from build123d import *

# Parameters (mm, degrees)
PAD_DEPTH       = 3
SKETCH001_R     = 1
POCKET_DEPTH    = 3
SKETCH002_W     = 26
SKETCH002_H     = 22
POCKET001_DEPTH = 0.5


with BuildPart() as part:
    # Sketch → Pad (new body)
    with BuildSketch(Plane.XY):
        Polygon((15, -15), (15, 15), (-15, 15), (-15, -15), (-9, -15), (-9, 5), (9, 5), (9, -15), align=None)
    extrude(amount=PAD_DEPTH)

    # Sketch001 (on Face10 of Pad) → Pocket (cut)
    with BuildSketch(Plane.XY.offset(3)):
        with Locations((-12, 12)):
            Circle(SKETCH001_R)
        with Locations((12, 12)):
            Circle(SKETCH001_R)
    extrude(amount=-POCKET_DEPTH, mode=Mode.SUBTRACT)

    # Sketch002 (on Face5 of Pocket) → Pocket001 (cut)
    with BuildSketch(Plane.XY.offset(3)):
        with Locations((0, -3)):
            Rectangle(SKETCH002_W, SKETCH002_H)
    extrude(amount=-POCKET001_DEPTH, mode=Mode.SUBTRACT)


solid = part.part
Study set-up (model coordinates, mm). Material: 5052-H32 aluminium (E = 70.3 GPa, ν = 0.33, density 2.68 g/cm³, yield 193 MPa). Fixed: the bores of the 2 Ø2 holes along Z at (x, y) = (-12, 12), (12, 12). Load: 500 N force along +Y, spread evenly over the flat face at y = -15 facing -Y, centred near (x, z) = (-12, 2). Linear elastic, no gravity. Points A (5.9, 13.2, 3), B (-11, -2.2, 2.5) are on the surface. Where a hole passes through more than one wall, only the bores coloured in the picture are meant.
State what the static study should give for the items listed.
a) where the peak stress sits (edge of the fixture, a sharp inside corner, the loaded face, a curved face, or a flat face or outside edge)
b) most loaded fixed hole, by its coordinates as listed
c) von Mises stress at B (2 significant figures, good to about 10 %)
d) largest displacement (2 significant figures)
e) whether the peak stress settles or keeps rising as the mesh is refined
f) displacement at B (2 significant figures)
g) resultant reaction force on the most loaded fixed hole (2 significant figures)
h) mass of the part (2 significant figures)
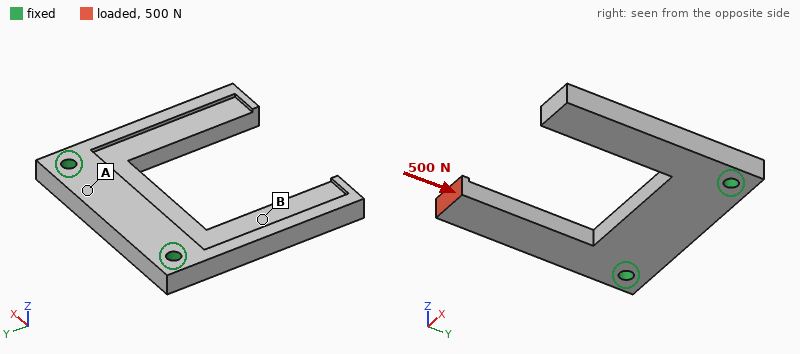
edge of the fixture
(-12, 12)
43 MPa
37 µm
keeps rising
9.9 µm
500 N
4.0 g
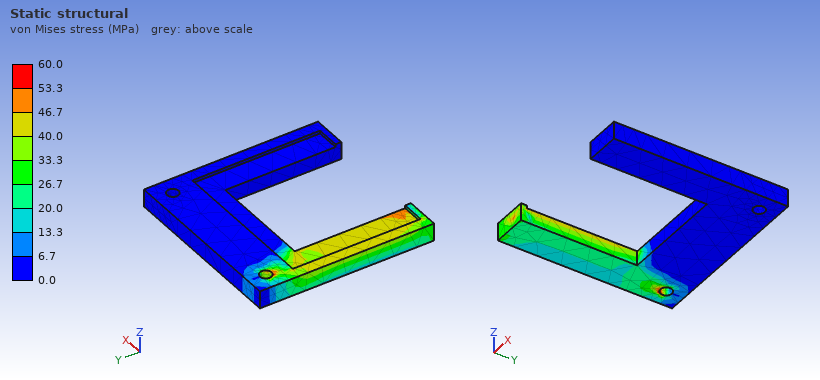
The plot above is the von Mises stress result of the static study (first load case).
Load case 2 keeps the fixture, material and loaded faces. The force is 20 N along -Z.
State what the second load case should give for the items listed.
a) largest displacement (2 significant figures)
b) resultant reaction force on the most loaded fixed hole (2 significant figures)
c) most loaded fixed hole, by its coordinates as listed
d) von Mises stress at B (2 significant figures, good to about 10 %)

0.15 mm
22 N
(-12, 12)
32 MPa
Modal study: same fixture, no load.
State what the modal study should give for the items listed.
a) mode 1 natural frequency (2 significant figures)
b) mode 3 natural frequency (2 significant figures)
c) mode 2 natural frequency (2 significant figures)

3500 Hz
8100 Hz
3600 Hz
